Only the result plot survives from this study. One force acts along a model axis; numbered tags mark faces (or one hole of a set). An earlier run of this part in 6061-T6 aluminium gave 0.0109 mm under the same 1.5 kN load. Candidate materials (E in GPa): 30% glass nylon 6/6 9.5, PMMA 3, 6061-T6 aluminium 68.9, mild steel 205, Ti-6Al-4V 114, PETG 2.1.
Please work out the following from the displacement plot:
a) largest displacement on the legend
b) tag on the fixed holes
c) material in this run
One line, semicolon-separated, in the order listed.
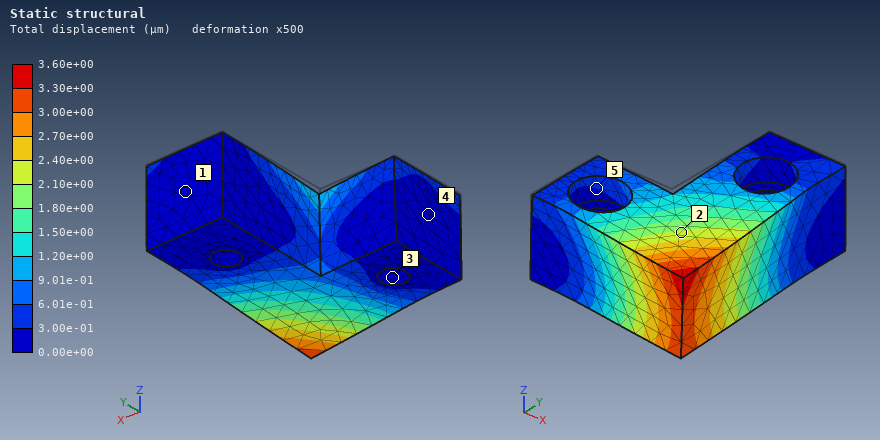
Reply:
3.60e+00 µm; 3; mild steel
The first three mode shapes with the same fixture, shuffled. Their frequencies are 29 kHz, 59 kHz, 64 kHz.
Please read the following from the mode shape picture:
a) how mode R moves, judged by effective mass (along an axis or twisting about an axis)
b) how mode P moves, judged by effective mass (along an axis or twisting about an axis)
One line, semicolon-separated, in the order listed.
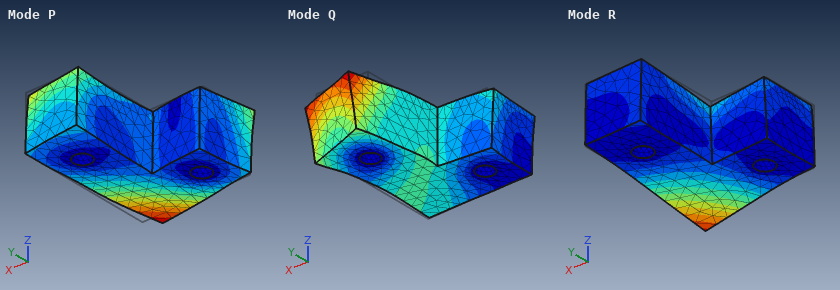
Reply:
along Z; along Y
